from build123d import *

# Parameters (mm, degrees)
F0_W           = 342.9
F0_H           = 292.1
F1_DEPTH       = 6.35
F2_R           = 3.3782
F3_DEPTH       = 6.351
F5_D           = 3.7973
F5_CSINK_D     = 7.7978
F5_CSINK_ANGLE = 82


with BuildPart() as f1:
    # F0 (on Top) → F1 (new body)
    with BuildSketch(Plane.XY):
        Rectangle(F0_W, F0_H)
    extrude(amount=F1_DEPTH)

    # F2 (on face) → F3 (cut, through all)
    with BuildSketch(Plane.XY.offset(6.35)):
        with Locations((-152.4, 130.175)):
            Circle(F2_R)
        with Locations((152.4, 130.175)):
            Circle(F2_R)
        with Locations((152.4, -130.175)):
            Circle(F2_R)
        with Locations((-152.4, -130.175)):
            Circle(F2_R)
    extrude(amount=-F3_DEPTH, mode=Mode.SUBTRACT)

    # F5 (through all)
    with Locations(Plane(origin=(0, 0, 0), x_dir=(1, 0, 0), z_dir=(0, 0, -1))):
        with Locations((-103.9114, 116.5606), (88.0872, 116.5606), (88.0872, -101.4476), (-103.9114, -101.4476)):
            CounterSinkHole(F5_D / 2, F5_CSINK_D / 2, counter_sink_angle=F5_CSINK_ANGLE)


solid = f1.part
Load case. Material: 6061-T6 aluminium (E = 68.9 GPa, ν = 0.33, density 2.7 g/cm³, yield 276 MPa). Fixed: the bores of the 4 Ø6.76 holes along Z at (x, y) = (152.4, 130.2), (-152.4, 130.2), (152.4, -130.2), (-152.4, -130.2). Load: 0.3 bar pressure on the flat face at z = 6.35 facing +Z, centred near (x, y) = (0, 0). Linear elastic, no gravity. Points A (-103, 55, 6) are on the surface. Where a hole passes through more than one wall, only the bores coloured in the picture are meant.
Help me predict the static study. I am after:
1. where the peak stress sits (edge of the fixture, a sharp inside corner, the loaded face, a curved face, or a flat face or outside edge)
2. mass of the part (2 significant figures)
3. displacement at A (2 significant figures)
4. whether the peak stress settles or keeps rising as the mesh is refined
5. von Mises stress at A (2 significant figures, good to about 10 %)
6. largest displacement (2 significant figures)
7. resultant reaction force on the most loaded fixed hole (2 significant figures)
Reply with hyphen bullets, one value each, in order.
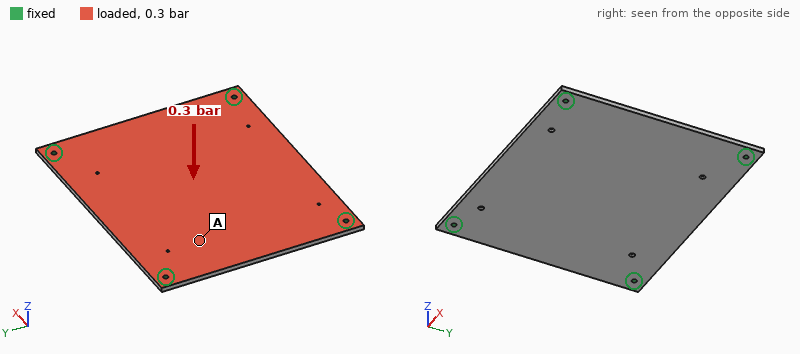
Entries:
- edge of the fixture
- 1.7 kg
- 0.62 mm
- keeps rising
- 13 MPa
- 1.1 mm
- 750 N
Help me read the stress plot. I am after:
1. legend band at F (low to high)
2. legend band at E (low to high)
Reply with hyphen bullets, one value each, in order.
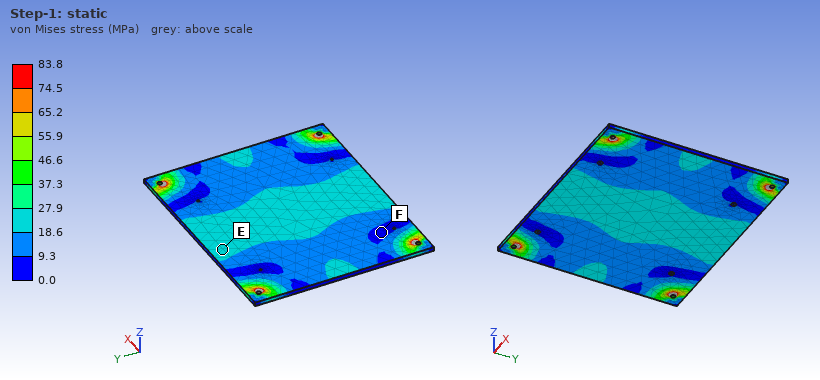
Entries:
- 0.0 to 9.3 MPa
- 18.6 to 27.9 MPa
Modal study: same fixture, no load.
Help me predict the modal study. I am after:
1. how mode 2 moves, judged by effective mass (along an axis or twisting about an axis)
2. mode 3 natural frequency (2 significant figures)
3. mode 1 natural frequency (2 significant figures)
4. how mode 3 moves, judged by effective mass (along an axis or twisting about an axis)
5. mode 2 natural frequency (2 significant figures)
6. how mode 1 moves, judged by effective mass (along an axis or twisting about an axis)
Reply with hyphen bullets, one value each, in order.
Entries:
- twisting about X
- 480 Hz
- 240 Hz
- twisting about Y
- 400 Hz
- along Z
